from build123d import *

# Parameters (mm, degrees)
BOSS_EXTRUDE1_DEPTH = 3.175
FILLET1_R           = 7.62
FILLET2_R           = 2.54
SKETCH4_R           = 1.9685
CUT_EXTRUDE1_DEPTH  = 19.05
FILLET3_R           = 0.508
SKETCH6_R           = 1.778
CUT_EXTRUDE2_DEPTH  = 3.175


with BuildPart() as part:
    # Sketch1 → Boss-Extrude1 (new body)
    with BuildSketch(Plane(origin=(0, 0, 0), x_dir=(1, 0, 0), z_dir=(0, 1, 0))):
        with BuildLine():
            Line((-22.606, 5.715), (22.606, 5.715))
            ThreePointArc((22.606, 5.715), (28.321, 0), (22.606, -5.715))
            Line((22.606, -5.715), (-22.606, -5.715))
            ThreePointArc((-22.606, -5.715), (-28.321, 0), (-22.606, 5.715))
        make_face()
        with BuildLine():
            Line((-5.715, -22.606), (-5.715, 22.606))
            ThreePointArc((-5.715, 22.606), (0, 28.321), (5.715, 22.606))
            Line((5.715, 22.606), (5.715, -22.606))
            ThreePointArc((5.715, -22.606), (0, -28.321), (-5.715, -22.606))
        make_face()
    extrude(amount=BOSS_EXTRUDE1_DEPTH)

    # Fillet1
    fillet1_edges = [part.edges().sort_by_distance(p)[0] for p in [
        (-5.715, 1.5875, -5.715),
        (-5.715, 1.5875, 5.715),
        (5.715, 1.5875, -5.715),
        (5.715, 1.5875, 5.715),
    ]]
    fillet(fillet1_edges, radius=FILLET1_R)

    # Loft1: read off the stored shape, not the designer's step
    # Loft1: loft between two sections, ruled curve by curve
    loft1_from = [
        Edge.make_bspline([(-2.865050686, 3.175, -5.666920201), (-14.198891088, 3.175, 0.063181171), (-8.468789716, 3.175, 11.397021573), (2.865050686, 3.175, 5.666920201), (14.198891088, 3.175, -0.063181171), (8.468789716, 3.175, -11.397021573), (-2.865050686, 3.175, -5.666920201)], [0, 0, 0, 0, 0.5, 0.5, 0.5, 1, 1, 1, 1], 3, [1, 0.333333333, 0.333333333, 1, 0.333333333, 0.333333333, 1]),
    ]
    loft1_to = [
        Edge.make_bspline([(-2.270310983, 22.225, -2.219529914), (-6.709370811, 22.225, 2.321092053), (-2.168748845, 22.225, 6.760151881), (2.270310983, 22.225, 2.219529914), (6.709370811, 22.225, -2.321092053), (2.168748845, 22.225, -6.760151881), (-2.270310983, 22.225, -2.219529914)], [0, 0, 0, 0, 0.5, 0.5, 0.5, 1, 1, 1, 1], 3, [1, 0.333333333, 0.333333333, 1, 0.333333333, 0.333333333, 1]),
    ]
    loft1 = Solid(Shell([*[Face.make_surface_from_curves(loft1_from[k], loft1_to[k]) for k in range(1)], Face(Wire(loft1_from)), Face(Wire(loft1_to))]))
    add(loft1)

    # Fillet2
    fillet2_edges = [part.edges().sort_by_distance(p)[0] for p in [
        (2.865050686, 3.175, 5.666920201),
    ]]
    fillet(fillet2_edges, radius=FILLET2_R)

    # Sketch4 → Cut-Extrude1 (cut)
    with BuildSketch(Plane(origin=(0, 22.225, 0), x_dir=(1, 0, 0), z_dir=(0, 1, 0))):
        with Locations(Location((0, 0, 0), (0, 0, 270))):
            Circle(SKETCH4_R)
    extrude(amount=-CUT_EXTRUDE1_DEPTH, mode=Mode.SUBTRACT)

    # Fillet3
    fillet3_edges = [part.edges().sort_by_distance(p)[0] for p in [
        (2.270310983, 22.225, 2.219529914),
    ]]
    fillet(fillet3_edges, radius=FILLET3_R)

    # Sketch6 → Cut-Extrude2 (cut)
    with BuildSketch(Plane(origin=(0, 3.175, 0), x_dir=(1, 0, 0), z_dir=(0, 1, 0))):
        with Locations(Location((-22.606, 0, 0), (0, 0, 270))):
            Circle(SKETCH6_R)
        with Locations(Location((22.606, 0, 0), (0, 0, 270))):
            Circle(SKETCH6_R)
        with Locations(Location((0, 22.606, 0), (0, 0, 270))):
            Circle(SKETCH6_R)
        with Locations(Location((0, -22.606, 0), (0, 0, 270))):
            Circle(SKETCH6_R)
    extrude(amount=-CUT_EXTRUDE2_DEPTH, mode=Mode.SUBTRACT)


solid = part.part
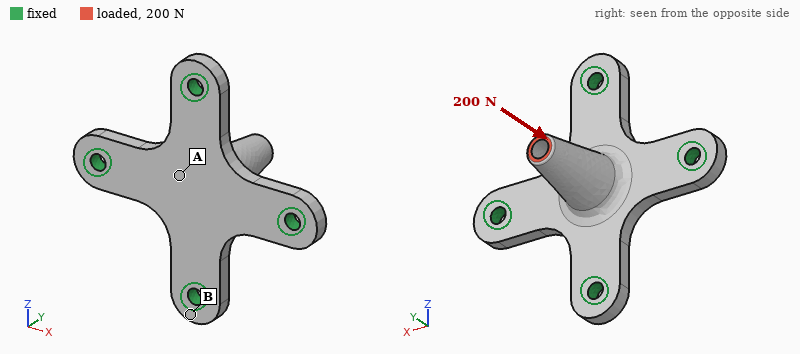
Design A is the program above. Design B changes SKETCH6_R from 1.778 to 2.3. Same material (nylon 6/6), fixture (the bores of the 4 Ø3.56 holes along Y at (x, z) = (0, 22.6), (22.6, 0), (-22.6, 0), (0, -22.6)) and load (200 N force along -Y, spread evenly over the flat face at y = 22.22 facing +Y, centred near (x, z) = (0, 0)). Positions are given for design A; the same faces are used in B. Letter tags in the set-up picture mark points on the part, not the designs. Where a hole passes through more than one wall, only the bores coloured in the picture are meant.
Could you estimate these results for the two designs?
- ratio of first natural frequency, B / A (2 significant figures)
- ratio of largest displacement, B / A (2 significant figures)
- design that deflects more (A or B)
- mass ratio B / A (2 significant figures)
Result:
1.1
0.91
A
0.98
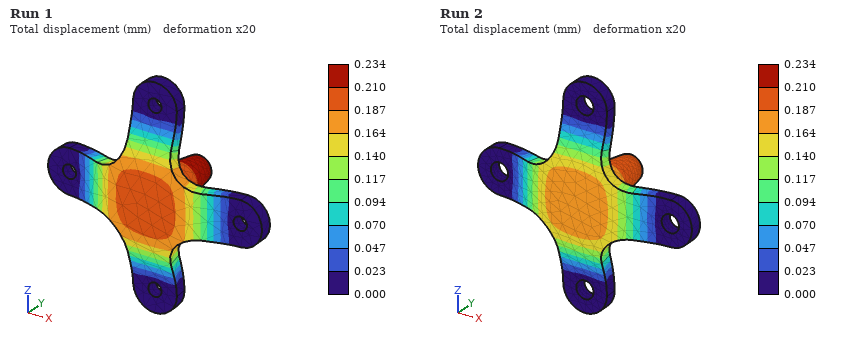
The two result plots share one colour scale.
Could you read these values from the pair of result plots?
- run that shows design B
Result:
Run 2
